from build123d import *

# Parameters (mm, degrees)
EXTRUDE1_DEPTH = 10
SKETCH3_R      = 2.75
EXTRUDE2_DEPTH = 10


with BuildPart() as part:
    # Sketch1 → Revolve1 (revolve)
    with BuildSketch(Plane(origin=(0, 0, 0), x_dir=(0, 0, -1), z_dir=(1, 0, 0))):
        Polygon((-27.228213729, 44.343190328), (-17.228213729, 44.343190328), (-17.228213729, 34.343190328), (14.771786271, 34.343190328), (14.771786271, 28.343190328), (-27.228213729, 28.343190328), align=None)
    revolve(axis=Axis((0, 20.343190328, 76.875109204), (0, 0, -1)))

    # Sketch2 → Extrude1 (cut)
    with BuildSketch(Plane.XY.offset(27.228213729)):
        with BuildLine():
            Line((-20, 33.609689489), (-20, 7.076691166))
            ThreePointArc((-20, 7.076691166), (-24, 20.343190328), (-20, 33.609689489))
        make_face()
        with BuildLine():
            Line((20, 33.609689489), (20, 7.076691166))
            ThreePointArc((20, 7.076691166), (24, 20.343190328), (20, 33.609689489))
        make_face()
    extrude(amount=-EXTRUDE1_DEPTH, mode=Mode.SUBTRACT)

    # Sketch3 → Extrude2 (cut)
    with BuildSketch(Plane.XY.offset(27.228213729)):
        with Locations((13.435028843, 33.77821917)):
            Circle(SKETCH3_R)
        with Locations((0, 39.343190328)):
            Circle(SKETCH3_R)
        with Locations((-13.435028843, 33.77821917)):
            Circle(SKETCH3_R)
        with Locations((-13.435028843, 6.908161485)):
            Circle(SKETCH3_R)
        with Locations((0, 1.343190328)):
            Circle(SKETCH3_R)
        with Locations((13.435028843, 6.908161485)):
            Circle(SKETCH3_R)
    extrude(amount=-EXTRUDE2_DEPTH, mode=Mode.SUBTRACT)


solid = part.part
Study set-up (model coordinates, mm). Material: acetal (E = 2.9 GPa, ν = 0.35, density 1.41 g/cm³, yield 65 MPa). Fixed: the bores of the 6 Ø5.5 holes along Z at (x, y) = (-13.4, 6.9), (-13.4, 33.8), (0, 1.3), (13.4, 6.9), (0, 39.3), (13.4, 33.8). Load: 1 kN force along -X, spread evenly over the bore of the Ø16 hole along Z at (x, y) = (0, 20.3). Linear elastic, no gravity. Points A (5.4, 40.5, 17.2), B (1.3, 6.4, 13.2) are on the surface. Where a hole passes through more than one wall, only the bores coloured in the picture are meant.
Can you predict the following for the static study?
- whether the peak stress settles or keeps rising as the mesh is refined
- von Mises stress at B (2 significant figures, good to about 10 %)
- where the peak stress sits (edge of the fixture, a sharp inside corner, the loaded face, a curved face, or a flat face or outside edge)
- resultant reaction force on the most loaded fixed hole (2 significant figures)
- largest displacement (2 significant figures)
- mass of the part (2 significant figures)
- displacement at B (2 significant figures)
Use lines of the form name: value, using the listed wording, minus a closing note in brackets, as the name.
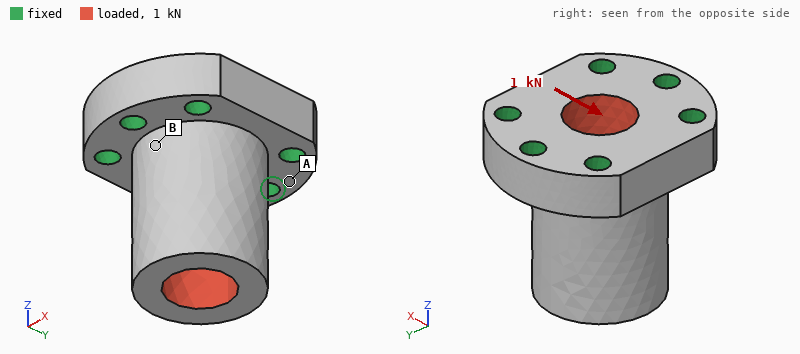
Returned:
whether the peak stress settles or keeps rising as the mesh is refined: keeps rising
von Mises stress at B: 3.5 MPa
where the peak stress sits: edge of the fixture
resultant reaction force on the most loaded fixed hole: 370 N
largest displacement: 0.15 mm
mass of the part: 37 g
displacement at B: 0.025 mm
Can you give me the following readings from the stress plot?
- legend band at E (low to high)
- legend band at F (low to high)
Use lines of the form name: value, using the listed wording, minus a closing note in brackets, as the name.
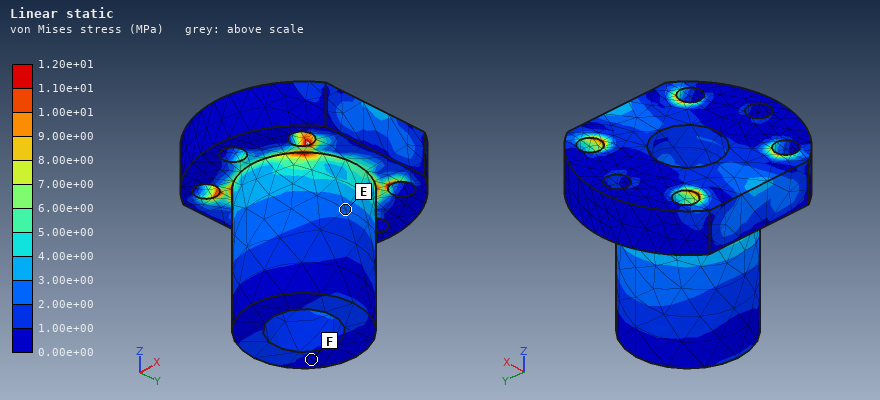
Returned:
legend band at E: 2.00e+00 to 3.00e+00 MPa
legend band at F: 0.00e+00 to 1.00e+00 MPa
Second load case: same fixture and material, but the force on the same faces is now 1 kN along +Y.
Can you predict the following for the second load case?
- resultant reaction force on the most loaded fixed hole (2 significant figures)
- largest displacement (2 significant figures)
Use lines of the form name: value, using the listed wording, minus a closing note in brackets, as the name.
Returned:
resultant reaction force on the most loaded fixed hole: 320 N
largest displacement: 0.13 mm
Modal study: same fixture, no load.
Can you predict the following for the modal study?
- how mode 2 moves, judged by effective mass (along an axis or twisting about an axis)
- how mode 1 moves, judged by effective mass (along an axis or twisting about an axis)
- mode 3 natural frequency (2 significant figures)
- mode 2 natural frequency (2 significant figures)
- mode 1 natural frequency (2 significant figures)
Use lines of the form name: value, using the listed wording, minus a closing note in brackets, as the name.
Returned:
how mode 2 moves, judged by effective mass: along Y
how mode 1 moves, judged by effective mass: along X
mode 3 natural frequency: 6200 Hz
mode 2 natural frequency: 3400 Hz
mode 1 natural frequency: 3100 Hz
